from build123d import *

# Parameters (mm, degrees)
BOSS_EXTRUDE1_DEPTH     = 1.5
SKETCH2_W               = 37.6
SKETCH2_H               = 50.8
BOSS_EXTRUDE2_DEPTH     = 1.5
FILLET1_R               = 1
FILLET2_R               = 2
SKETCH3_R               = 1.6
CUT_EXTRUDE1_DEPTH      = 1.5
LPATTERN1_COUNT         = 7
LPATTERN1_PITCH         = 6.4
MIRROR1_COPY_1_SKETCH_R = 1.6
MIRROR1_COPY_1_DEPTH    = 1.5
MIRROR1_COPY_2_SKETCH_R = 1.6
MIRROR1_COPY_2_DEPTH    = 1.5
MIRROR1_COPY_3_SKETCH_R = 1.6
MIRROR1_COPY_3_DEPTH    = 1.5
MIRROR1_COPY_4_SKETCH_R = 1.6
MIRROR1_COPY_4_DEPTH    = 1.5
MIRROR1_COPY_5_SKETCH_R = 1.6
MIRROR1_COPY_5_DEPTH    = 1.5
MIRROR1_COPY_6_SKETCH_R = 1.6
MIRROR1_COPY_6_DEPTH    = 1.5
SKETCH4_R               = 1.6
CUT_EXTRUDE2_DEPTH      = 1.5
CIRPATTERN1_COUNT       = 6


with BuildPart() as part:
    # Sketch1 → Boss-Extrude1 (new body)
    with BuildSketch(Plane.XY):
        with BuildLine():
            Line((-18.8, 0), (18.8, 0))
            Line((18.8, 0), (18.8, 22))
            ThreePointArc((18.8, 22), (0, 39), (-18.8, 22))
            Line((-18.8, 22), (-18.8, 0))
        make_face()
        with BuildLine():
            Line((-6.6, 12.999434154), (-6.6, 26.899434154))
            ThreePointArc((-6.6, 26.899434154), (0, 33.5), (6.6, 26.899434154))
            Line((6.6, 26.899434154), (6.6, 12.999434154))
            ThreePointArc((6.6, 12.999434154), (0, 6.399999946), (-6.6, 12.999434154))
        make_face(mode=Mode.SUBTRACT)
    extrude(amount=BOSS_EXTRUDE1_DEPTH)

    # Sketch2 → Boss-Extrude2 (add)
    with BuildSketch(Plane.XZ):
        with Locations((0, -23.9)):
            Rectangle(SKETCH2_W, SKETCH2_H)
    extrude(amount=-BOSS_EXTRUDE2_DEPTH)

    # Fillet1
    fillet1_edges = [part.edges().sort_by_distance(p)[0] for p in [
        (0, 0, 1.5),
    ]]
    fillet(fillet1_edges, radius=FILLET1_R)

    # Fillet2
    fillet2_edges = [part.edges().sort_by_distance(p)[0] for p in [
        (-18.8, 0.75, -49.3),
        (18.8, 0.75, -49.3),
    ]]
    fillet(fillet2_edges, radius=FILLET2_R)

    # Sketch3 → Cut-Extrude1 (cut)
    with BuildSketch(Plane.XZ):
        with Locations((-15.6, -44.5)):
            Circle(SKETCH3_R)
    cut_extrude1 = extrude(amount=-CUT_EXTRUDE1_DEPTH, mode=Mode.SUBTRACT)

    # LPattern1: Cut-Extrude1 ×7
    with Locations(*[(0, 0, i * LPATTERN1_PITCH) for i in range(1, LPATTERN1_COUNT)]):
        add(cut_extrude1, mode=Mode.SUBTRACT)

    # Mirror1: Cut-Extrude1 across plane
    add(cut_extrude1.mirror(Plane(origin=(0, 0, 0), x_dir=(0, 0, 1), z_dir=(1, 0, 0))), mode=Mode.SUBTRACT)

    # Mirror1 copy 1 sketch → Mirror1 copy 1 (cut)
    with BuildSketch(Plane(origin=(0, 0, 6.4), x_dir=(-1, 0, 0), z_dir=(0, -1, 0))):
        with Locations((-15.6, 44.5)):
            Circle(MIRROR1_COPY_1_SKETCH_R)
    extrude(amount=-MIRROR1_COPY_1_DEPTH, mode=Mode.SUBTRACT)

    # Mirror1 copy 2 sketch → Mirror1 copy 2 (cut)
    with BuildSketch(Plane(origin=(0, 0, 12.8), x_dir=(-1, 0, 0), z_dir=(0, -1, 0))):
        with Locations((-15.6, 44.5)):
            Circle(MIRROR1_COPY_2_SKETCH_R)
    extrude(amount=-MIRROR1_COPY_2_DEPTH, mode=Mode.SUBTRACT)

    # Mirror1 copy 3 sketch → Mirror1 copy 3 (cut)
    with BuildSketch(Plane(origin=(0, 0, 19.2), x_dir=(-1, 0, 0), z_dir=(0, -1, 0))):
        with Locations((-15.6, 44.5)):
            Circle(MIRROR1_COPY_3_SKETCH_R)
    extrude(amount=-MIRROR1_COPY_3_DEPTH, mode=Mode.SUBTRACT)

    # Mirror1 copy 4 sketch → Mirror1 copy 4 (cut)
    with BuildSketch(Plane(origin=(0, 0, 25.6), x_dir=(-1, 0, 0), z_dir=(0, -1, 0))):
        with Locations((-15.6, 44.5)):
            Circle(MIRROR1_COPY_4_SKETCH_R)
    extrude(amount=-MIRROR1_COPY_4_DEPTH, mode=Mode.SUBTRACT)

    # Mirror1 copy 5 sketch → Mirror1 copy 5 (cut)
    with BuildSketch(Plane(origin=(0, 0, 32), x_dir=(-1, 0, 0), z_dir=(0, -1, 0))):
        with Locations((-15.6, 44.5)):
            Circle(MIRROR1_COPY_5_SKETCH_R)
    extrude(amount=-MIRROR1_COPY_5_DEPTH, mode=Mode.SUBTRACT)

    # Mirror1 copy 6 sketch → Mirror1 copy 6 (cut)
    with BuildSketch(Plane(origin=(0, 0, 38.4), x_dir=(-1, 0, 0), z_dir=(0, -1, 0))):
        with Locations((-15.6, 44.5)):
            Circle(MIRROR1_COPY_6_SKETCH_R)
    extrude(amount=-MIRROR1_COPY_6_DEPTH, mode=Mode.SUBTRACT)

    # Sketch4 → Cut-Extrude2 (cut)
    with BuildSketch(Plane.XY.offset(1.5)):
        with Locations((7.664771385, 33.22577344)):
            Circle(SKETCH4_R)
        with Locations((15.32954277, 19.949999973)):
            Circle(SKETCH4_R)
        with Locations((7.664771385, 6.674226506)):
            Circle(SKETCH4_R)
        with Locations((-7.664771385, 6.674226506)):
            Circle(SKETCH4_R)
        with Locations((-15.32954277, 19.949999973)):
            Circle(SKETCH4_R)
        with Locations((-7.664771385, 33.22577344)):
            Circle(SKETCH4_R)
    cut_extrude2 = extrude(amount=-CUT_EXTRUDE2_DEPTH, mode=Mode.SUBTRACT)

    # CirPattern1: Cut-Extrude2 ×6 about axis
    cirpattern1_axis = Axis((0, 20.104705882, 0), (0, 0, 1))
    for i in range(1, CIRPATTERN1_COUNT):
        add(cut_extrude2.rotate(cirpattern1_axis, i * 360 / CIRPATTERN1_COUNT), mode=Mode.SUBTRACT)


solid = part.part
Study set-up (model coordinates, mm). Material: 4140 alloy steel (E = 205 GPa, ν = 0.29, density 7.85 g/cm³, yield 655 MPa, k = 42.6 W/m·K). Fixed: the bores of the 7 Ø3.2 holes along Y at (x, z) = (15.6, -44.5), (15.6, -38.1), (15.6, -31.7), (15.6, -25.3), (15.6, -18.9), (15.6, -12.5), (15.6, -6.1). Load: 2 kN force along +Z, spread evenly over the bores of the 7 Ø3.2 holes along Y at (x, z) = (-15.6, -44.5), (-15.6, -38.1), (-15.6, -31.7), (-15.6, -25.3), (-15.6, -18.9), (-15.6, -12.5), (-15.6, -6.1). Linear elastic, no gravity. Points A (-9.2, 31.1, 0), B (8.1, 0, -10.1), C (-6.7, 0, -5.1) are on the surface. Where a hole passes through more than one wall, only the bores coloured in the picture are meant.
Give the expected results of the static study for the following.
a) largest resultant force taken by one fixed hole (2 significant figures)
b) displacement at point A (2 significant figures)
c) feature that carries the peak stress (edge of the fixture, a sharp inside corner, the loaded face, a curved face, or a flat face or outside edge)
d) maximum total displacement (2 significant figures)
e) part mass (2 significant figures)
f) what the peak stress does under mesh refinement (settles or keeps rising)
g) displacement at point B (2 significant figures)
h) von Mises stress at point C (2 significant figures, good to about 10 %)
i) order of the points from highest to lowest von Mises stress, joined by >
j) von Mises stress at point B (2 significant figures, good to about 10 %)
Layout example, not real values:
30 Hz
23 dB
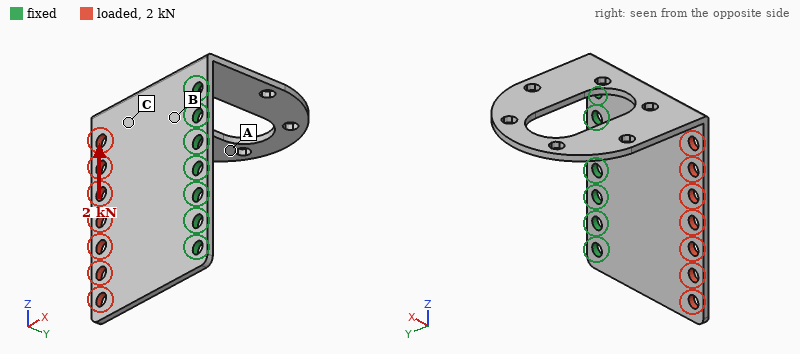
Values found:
1.3 kN
16 µm
edge of the fixture
25 µm
31 g
keeps rising
4.0 µm
33 MPa
B > C > A
74 MPa
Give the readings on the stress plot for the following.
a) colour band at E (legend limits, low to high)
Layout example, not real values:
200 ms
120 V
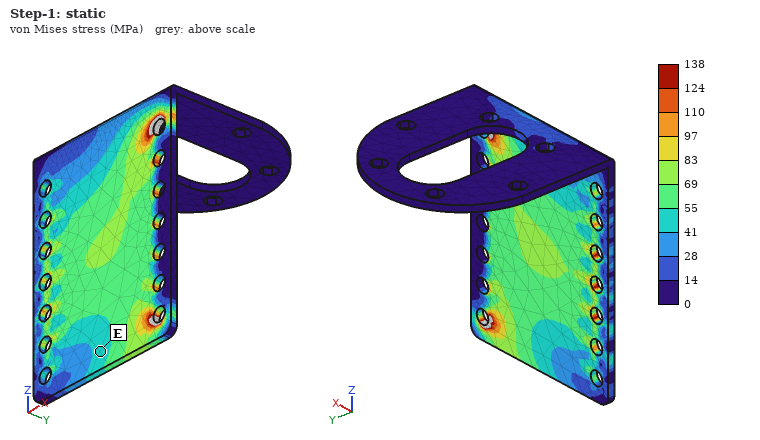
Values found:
41 to 55 MPa
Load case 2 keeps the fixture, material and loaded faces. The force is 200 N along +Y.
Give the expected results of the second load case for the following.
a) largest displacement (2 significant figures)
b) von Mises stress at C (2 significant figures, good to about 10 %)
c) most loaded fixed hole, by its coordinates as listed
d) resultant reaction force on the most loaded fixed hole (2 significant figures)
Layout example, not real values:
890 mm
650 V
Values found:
0.58 mm
110 MPa
(15.6, -6.1)
54 N
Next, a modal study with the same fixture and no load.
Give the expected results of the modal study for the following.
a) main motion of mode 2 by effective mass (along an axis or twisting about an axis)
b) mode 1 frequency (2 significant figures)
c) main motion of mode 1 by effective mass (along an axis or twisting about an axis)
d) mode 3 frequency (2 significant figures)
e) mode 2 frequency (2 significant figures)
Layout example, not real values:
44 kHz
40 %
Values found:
along Y
700 Hz
along Z
1600 Hz
940 Hz
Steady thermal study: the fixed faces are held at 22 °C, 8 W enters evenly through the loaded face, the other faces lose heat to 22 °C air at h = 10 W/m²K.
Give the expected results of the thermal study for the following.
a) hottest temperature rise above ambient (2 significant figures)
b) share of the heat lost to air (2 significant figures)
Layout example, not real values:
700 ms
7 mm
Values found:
73 K
19 %
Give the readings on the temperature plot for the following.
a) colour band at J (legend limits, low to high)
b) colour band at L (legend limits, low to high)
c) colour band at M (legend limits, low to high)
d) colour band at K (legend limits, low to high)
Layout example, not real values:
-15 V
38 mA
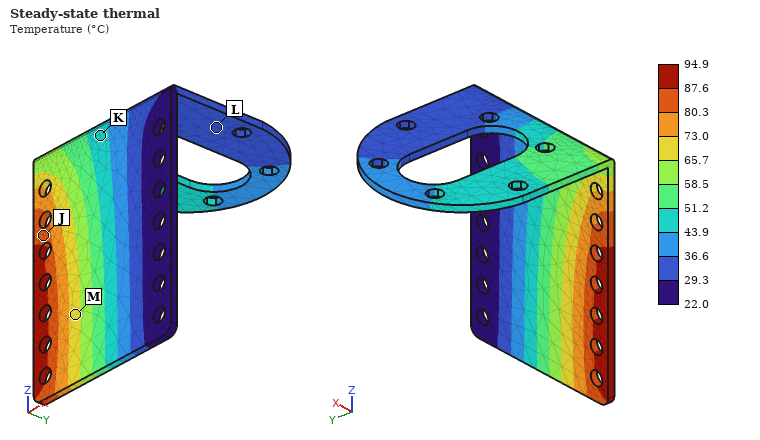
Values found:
80.3 to 87.6 °C
29.3 to 36.6 °C
65.7 to 73.0 °C
43.9 to 51.2 °C
